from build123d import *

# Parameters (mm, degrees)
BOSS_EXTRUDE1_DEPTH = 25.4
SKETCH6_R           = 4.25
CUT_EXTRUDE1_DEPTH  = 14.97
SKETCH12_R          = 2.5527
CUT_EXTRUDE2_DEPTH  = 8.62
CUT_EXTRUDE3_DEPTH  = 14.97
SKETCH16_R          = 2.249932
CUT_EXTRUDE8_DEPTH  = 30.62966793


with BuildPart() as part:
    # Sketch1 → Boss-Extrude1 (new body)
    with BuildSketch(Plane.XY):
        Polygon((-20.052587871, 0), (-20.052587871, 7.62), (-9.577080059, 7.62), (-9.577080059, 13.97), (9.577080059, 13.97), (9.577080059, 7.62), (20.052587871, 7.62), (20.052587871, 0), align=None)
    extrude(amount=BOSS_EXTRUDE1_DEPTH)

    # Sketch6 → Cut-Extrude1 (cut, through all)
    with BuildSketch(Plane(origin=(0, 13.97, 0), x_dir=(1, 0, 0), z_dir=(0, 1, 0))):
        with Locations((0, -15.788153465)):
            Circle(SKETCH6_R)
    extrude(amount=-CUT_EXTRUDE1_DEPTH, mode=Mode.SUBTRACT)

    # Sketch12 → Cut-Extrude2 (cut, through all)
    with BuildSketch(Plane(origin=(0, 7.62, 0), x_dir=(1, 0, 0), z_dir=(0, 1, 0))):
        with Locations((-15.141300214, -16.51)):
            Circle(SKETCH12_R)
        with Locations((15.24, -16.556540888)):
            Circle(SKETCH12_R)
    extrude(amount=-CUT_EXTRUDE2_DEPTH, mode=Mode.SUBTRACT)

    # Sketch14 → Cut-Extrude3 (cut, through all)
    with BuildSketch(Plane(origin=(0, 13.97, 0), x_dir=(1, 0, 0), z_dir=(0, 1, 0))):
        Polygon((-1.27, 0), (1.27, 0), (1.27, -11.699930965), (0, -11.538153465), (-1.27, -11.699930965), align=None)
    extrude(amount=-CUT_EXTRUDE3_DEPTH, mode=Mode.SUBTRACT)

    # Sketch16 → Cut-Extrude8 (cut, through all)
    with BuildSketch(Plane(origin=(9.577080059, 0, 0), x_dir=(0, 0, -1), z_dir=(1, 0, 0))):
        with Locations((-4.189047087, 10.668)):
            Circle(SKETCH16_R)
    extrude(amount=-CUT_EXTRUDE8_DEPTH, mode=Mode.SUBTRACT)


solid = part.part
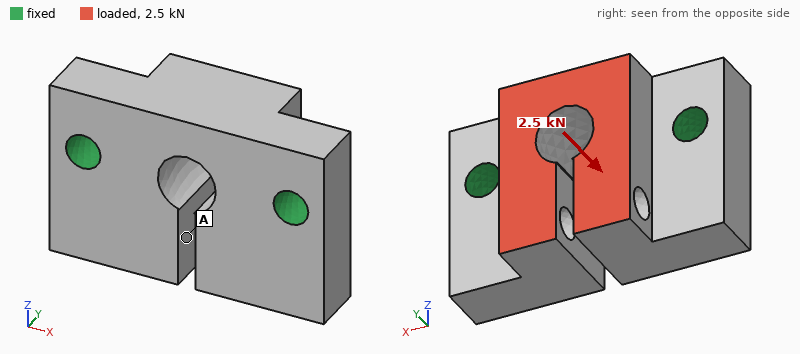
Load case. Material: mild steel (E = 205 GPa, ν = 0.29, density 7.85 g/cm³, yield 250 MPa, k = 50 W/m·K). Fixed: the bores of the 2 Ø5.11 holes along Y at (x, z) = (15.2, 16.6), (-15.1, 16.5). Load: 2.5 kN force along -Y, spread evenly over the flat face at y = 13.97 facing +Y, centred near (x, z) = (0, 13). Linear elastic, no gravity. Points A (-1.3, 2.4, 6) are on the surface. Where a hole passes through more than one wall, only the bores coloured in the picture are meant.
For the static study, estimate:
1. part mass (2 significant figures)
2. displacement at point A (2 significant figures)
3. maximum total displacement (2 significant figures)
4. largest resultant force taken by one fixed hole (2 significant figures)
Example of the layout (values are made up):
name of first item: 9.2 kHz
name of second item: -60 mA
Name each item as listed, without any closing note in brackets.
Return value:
part mass: 71 g
displacement at point A: 6.1 µm
maximum total displacement: 9.0 µm
largest resultant force taken by one fixed hole: 1.3 kN
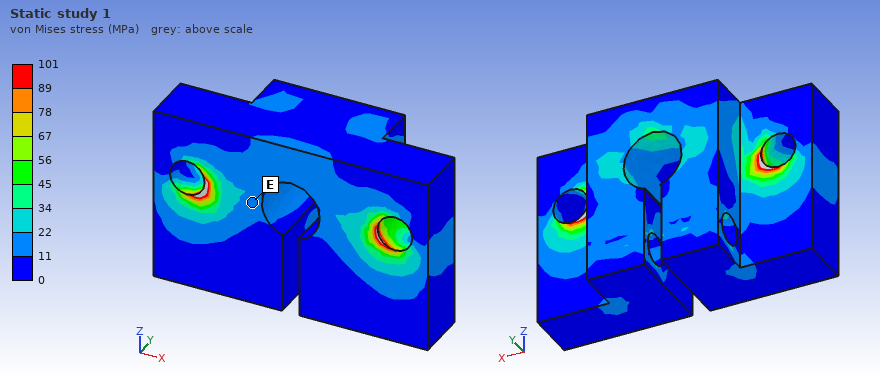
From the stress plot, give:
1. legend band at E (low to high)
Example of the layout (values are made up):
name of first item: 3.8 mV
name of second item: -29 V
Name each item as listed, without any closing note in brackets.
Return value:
legend band at E: 11 to 22 MPa
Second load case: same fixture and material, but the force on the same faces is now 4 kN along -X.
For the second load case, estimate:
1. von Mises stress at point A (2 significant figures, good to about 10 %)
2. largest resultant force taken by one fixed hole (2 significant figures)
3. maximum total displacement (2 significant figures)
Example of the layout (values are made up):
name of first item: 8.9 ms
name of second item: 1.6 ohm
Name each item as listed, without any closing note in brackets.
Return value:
von Mises stress at point A: 13 MPa
largest resultant force taken by one fixed hole: 2.3 kN
maximum total displacement: 18 µm
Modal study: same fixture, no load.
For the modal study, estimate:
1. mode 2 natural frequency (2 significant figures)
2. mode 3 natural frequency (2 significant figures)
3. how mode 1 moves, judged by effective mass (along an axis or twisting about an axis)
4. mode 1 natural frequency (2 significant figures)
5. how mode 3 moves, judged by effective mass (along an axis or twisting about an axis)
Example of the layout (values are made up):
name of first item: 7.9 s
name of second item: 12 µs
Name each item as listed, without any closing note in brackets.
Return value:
mode 2 natural frequency: 16 kHz
mode 3 natural frequency: 17 kHz
how mode 1 moves, judged by effective mass: along Y
mode 1 natural frequency: 15 kHz
how mode 3 moves, judged by effective mass: along Z
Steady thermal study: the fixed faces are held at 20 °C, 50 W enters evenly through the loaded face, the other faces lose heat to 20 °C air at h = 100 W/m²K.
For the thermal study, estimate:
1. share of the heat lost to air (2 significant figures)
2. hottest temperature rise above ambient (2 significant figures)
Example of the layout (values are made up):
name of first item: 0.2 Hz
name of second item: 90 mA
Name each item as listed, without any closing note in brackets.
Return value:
share of the heat lost to air: 16 %
hottest temperature rise above ambient: 55 K
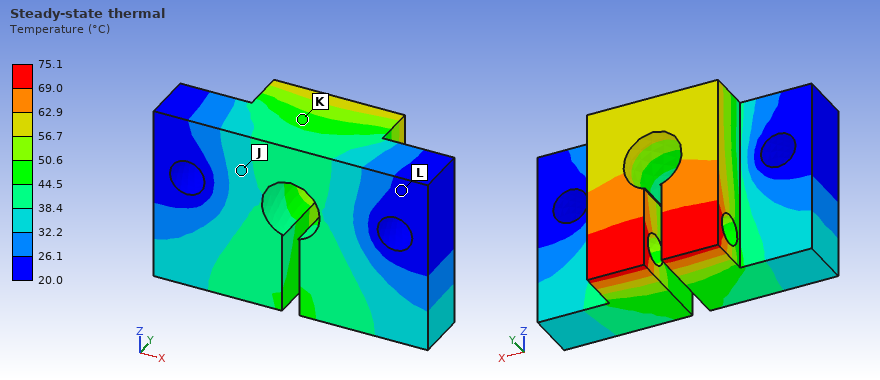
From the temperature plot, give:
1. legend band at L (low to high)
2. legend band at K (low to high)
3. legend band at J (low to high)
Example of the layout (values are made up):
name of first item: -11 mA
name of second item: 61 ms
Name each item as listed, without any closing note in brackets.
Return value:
legend band at L: 20.0 to 26.1 °C
legend band at K: 44.5 to 50.6 °C
legend band at J: 32.2 to 38.4 °C
